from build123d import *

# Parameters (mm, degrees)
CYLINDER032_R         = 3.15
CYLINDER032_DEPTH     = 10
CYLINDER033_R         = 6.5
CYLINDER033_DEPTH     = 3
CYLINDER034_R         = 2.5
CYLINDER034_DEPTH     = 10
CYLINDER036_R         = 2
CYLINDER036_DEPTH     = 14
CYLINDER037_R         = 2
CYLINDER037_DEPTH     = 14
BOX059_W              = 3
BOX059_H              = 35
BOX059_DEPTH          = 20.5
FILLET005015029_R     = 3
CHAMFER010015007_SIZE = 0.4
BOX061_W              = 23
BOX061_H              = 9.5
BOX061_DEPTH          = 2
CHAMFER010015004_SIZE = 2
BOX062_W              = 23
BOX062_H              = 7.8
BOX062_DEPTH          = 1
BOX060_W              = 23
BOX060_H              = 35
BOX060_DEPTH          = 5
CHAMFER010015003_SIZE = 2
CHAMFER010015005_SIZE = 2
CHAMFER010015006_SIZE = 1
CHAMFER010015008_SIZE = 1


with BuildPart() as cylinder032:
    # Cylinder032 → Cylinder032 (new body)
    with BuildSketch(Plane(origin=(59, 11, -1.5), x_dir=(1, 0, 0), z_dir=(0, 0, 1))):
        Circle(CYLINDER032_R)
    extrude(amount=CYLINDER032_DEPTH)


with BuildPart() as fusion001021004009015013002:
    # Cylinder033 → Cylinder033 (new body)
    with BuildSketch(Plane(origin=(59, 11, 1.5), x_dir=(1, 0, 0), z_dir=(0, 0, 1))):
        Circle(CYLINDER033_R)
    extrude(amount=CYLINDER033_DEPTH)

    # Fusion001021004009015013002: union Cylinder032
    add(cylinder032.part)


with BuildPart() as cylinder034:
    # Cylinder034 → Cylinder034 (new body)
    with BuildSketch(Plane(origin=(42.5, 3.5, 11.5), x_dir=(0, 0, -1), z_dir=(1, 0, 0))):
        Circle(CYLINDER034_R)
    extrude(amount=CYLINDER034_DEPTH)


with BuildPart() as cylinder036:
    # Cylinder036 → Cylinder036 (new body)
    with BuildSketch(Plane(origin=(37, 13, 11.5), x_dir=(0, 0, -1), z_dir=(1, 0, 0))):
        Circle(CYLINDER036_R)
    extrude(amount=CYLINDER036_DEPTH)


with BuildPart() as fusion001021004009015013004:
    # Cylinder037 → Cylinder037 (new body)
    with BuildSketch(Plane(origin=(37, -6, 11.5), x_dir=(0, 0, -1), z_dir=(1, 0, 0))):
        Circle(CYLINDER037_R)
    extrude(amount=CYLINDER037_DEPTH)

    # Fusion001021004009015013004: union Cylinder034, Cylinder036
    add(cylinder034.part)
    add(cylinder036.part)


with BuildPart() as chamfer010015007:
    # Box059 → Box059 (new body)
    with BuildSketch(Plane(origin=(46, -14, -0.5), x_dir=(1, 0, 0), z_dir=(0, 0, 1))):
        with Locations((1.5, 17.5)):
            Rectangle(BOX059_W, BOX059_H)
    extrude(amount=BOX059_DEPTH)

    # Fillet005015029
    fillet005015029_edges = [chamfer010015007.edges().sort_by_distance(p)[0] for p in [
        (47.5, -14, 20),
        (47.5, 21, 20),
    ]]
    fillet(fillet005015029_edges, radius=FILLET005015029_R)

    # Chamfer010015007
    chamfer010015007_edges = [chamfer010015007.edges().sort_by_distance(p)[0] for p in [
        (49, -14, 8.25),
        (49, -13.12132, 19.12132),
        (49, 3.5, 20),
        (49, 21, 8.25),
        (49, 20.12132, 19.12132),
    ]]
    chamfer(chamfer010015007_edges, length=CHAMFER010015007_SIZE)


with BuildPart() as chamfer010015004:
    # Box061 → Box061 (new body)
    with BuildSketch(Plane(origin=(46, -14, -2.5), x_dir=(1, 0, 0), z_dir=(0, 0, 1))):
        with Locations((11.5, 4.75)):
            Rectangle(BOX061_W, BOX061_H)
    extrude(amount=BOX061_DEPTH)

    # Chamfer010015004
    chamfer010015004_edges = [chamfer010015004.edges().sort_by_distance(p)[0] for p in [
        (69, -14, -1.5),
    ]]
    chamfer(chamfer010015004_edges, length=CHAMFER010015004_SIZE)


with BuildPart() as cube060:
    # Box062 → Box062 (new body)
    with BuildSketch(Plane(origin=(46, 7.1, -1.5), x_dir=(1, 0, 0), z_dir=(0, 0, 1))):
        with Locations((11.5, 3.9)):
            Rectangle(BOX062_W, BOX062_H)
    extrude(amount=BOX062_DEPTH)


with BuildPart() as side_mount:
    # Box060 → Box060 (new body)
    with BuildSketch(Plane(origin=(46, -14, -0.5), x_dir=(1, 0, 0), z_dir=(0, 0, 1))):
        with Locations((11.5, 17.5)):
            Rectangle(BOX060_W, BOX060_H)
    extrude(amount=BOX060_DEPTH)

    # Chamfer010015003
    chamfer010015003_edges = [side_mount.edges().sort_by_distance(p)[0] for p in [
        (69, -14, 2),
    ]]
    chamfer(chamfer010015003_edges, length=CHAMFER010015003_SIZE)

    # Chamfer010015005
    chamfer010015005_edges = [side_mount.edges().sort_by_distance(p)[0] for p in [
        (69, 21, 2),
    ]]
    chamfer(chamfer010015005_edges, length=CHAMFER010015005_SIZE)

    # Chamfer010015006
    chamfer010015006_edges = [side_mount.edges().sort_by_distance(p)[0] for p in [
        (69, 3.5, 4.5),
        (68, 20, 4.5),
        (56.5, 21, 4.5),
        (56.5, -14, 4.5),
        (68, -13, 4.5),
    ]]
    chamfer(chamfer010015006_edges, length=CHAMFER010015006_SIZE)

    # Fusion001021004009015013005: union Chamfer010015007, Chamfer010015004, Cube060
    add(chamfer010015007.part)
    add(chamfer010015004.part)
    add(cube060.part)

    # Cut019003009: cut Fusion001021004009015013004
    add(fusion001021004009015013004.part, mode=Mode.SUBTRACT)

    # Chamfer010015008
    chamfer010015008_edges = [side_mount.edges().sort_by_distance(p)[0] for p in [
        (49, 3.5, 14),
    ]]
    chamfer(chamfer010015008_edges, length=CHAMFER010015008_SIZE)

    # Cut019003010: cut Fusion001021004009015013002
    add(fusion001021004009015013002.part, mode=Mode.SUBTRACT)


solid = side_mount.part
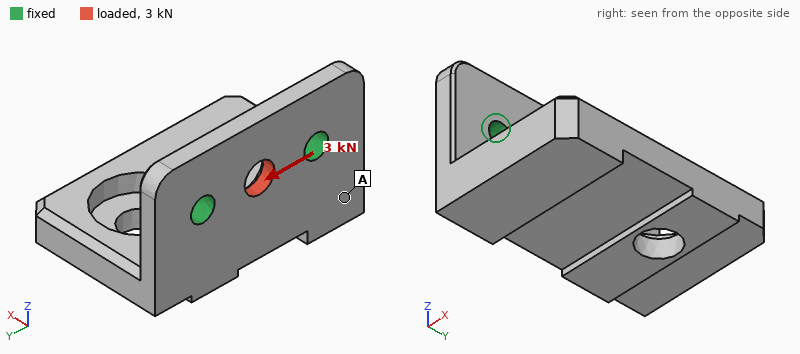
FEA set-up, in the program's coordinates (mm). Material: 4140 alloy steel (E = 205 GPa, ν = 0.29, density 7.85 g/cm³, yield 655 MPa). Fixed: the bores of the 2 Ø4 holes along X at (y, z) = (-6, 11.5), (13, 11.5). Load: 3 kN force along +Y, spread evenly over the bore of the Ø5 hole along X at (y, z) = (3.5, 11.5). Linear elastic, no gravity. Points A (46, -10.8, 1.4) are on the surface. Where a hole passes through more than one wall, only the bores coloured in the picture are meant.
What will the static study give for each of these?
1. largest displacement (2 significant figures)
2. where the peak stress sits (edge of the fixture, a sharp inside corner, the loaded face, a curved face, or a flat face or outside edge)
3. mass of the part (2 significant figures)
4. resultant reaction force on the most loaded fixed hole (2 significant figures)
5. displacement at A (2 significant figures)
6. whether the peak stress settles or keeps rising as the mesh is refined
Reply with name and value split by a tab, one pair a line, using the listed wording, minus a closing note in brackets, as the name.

largest displacement	2.6 µm
where the peak stress sits	a sharp inside corner
mass of the part	44 g
resultant reaction force on the most loaded fixed hole	1.5 kN
displacement at A	0.79 µm
whether the peak stress settles or keeps rising as the mesh is refined	keeps rising
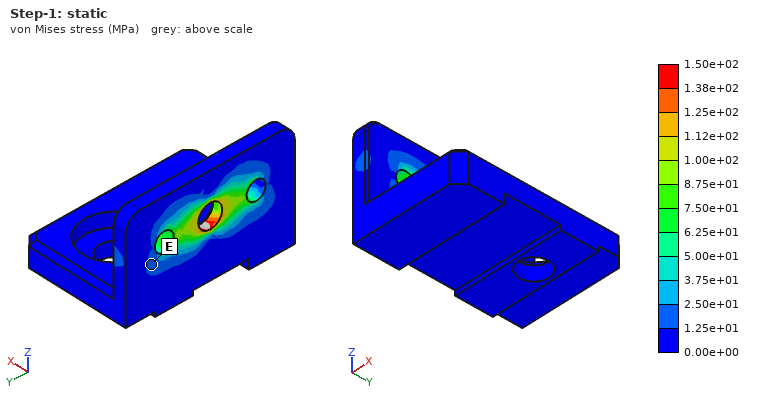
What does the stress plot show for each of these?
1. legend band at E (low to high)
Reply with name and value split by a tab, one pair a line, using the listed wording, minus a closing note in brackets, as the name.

legend band at E	1.25e+01 to 2.50e+01 MPa
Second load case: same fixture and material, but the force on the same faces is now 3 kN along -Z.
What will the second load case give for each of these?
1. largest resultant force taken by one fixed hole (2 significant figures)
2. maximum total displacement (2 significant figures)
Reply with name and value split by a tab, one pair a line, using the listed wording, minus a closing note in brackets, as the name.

largest resultant force taken by one fixed hole	1.5 kN
maximum total displacement	5.0 µm
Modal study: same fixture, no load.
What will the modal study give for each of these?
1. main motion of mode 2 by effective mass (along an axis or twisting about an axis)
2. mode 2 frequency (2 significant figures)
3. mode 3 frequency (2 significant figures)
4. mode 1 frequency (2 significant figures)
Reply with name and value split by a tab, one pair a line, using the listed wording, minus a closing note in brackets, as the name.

main motion of mode 2 by effective mass	along Y
mode 2 frequency	6700 Hz
mode 3 frequency	12 kHz
mode 1 frequency	2900 Hz
